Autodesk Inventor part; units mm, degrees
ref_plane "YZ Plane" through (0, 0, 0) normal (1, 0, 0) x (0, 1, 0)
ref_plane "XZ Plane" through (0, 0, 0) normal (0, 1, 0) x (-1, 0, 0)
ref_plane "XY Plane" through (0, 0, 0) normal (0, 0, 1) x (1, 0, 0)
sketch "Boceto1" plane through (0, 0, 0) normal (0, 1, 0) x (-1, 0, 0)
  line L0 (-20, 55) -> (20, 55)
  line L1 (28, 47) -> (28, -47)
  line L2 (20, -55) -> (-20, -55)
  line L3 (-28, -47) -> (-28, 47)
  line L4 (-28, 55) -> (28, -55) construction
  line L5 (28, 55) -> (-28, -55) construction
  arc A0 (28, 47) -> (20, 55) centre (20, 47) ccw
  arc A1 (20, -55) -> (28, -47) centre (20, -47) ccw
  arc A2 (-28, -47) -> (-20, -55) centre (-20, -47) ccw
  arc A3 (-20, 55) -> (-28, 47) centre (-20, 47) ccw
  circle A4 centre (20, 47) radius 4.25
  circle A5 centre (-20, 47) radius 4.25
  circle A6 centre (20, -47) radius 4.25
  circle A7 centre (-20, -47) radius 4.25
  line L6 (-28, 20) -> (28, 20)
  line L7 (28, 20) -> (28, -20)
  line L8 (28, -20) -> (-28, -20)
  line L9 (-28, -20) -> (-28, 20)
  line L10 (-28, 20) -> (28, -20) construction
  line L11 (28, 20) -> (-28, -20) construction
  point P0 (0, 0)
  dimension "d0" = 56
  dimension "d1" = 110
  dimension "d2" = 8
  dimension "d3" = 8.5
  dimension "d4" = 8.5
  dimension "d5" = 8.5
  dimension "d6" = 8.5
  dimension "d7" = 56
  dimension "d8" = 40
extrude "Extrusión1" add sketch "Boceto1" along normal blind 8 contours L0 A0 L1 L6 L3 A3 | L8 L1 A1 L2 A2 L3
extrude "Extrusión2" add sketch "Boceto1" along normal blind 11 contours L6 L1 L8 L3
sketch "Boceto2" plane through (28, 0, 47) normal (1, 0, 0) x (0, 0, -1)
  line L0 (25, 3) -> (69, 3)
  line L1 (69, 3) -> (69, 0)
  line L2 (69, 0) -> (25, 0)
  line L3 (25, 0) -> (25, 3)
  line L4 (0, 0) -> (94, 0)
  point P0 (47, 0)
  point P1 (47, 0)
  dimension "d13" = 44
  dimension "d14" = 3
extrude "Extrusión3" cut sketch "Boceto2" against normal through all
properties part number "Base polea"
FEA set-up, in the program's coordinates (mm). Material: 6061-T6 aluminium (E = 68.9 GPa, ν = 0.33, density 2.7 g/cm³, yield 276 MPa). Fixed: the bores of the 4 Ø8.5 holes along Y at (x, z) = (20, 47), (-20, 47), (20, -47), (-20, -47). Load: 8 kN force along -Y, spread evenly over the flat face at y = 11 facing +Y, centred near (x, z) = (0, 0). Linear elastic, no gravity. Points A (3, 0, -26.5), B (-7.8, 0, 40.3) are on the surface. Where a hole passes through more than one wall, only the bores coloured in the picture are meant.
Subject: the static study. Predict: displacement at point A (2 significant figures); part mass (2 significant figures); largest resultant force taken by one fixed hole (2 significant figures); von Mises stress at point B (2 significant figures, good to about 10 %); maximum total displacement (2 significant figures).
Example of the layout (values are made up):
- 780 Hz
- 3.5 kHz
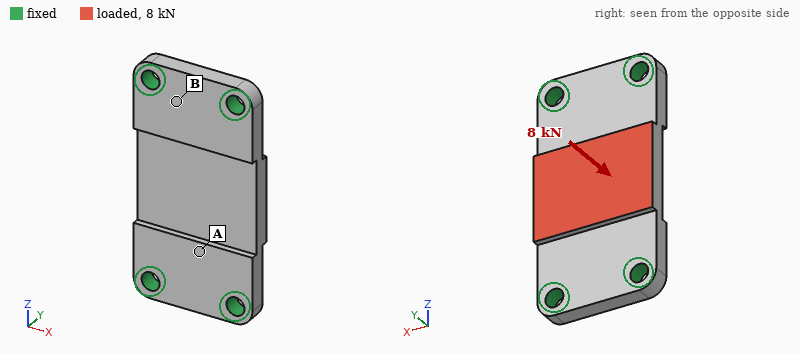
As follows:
- 0.079 mm
- 130 g
- 4.1 kN
- 60 MPa
- 0.16 mm
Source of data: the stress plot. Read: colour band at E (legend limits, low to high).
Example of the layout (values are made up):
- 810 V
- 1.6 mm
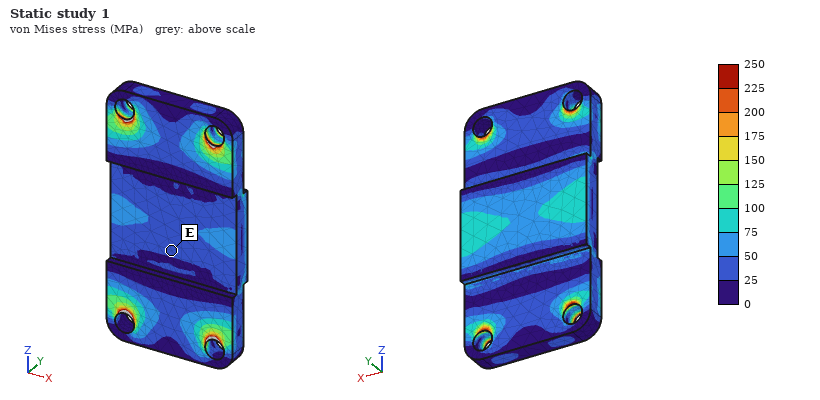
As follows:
- 25 to 50 MPa
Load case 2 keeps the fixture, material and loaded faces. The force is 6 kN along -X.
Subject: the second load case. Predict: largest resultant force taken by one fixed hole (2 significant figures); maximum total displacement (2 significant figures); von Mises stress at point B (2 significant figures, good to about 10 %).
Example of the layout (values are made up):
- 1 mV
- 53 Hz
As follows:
- 2.5 kN
- 48 µm
- 7.0 MPa
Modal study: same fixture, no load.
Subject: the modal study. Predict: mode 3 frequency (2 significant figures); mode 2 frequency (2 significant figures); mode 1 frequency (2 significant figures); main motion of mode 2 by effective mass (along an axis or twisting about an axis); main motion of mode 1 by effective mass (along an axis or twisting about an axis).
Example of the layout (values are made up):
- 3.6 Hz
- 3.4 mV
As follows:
- 10 kHz
- 6900 Hz
- 5100 Hz
- twisting about Z
- along Y
